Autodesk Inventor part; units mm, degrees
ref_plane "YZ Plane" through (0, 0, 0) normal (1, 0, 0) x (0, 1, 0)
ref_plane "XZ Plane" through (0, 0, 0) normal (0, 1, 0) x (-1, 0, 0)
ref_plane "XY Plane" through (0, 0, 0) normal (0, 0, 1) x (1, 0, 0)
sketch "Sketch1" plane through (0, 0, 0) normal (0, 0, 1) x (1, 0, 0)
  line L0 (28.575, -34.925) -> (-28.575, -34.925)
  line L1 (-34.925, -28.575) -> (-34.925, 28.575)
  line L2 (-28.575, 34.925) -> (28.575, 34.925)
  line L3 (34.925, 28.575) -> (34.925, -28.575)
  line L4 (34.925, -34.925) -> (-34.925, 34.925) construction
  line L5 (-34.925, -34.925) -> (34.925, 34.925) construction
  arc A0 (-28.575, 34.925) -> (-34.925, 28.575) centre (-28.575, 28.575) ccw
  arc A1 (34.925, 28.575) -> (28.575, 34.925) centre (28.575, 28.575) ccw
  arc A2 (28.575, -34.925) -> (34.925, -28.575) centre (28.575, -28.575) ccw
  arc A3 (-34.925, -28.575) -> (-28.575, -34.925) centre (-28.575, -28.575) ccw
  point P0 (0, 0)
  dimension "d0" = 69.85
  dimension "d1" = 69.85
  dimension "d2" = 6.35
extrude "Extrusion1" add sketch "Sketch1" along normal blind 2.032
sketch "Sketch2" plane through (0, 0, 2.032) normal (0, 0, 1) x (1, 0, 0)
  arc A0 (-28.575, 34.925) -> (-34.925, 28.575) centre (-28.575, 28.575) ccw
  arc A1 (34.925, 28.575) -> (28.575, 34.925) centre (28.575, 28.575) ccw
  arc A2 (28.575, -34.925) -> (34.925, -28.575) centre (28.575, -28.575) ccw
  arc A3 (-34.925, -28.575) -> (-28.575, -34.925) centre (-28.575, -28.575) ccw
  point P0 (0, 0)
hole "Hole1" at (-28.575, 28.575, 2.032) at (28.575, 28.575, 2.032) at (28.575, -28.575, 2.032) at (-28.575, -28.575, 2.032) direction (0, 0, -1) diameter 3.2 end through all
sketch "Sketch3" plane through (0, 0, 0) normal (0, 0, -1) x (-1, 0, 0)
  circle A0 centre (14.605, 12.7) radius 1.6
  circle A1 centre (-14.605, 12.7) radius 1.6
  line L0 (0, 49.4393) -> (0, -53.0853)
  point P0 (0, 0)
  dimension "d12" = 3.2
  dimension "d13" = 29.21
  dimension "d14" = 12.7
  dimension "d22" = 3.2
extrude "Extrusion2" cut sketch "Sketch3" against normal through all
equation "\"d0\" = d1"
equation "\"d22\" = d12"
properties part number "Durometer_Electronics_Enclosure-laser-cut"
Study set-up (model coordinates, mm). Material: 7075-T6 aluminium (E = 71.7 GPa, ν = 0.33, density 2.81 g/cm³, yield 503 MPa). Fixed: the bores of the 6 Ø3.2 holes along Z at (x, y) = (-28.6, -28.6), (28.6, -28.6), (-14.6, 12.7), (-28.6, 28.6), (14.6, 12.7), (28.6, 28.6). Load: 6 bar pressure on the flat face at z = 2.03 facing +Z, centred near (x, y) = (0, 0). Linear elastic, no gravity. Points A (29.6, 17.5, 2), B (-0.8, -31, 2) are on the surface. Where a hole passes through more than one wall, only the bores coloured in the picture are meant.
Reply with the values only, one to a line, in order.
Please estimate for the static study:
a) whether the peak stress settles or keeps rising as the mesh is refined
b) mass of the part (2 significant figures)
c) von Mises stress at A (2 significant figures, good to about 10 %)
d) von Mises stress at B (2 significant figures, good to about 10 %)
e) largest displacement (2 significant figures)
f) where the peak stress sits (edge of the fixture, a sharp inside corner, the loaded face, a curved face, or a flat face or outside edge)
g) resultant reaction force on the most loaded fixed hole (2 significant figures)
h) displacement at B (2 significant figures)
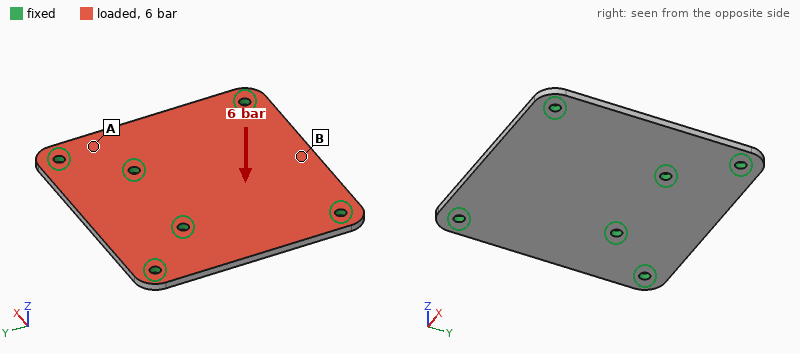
keeps rising
27 g
36 MPa
110 MPa
0.33 mm
edge of the fixture
690 N
0.32 mm
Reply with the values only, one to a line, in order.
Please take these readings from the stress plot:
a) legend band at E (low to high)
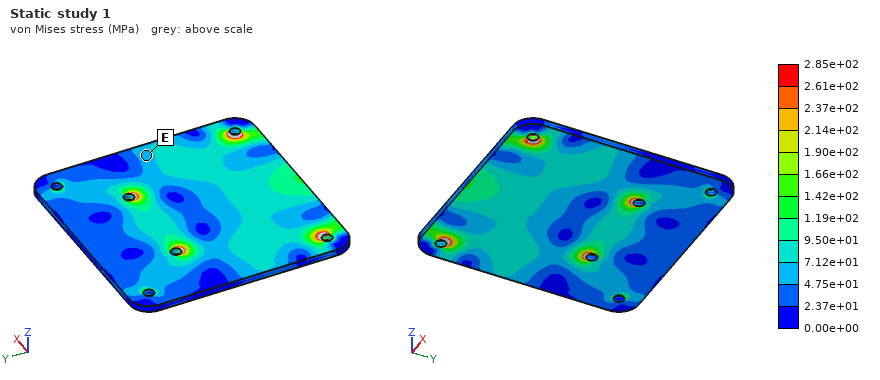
4.75e+01 to 7.12e+01 MPa
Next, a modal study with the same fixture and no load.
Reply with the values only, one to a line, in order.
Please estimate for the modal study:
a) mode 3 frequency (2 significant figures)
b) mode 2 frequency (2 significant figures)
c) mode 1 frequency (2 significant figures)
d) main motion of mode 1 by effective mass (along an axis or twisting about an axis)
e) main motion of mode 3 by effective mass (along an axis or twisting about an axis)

4900 Hz
4700 Hz
3400 Hz
along Z
twisting about Y
